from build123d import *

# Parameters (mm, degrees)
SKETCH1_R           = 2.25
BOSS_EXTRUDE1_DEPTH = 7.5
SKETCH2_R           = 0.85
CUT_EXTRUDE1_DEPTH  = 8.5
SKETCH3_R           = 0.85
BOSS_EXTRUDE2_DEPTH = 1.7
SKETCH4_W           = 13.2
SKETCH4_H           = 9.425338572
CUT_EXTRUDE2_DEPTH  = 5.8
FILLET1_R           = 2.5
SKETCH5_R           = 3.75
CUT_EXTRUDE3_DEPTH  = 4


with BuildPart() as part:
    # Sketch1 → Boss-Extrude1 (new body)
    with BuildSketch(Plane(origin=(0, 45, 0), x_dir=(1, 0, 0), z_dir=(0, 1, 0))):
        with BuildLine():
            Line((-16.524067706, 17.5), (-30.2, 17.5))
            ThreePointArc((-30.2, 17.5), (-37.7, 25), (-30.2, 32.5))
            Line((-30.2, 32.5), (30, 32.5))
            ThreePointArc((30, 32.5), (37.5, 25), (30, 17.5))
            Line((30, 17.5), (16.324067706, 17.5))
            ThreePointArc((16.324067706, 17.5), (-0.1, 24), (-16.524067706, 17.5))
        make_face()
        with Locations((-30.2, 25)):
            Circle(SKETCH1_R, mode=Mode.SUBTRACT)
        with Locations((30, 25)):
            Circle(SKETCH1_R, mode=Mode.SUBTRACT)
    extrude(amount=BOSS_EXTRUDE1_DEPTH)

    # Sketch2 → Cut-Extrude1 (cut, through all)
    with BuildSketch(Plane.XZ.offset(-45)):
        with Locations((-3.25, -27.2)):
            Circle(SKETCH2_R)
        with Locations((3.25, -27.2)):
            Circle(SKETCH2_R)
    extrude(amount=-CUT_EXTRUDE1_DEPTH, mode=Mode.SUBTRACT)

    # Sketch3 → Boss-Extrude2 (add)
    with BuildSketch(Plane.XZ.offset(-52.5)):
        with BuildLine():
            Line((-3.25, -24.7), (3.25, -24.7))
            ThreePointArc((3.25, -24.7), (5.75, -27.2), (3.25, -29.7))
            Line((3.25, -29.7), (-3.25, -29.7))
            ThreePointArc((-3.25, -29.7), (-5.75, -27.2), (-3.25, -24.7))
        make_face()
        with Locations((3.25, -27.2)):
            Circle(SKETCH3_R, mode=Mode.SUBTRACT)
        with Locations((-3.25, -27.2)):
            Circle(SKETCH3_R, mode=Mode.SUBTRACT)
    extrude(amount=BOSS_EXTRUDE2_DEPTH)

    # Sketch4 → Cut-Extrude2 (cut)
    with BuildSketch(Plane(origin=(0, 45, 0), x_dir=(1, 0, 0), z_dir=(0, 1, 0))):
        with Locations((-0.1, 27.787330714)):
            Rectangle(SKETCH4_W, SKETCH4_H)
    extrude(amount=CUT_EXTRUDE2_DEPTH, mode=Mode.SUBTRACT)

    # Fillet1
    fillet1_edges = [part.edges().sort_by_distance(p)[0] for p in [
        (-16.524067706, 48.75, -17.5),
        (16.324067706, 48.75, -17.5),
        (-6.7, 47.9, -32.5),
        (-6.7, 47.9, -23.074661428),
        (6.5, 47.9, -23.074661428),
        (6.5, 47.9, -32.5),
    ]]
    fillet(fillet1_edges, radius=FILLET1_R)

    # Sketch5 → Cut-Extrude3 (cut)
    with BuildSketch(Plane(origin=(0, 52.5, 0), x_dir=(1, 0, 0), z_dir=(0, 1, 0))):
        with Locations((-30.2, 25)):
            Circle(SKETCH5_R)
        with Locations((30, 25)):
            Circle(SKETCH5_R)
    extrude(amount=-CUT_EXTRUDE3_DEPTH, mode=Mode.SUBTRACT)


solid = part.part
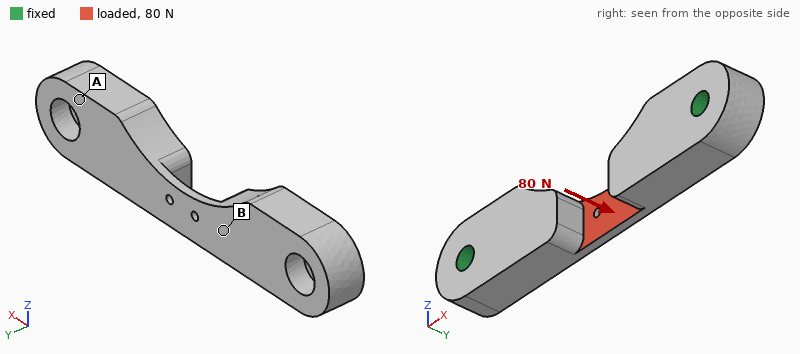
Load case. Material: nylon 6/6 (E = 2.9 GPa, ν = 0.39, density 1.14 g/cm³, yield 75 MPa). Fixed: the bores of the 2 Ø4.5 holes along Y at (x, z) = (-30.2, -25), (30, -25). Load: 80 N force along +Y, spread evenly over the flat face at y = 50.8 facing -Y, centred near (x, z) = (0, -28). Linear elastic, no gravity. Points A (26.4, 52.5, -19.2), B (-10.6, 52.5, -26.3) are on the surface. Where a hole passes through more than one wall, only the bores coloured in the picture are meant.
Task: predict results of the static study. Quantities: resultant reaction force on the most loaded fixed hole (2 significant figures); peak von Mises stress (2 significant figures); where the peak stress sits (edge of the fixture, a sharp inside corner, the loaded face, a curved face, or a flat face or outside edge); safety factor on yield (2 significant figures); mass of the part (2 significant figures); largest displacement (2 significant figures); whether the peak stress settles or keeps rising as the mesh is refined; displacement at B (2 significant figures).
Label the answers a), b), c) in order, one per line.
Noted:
a) 100 N
b) 33 MPa
c) a curved face
d) 2.3
e) 6.6 g
f) 0.29 mm
g) settles
h) 0.13 mm
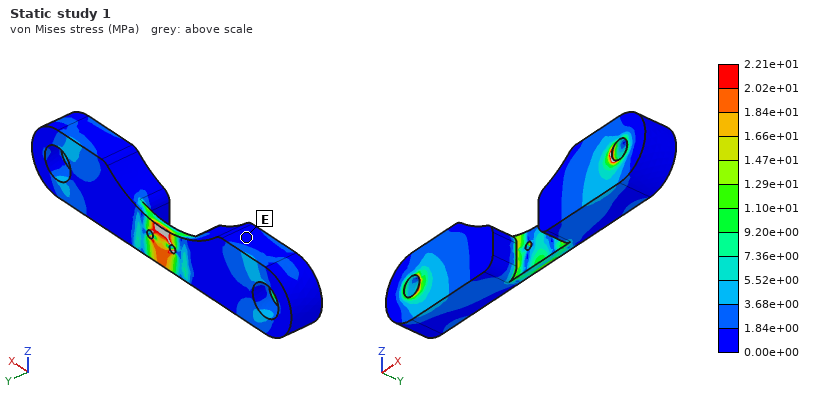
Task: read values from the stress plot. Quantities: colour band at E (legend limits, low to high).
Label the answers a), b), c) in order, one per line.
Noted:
a) 0.00e+00 to 1.84e+00 MPa
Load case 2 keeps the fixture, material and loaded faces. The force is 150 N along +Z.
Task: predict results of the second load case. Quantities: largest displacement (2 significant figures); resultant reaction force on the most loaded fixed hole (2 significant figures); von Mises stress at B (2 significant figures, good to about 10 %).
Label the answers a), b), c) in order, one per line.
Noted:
a) 0.28 mm
b) 86 N
c) 4.6 MPa
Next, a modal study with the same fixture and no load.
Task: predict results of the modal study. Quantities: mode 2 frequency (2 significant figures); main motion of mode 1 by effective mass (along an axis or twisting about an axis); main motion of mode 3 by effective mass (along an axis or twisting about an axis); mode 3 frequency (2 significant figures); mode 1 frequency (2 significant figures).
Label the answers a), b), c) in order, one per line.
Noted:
a) 3000 Hz
b) along Y
c) along Z
d) 3600 Hz
e) 2700 Hz
